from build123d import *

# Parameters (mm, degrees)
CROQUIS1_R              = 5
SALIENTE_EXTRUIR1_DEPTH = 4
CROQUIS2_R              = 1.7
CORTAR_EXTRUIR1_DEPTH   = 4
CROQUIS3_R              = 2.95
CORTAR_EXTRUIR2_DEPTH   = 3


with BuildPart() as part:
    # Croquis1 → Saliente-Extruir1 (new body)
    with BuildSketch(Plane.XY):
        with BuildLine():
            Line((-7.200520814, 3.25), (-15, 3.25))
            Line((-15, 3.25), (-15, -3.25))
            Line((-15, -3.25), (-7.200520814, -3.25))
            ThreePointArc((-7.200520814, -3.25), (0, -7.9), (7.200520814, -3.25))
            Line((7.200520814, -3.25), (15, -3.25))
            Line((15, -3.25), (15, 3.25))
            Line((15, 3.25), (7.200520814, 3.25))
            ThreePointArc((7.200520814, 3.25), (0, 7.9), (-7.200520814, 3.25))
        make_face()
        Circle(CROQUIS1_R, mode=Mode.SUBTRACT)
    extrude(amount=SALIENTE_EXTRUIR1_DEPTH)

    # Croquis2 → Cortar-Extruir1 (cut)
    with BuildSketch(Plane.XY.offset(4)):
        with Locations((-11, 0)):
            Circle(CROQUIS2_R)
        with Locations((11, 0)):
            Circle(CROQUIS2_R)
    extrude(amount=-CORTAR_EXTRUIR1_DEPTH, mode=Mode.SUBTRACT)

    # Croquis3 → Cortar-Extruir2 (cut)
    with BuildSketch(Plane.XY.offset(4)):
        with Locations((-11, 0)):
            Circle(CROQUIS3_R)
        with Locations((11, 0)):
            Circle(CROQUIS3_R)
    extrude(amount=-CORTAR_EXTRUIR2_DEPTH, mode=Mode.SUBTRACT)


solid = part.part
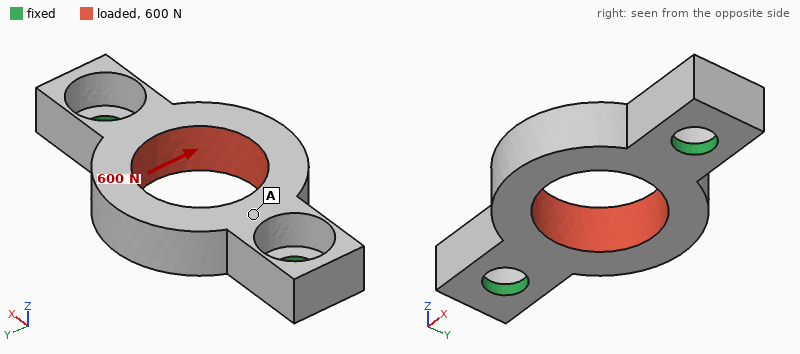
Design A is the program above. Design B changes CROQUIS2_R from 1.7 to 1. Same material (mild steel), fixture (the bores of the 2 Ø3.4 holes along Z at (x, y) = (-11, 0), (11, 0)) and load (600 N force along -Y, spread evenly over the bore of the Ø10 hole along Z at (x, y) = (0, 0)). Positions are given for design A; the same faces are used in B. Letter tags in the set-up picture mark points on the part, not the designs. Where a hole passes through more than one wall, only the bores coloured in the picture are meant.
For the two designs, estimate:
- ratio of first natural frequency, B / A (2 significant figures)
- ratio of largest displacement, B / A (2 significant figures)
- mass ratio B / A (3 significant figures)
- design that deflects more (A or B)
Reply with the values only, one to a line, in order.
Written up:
0.72
2.0
1.02
B
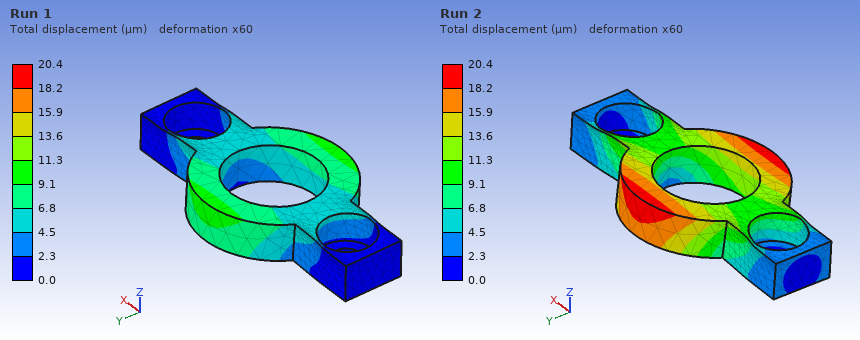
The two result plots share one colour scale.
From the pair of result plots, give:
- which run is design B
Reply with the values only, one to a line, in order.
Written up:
Run 2
